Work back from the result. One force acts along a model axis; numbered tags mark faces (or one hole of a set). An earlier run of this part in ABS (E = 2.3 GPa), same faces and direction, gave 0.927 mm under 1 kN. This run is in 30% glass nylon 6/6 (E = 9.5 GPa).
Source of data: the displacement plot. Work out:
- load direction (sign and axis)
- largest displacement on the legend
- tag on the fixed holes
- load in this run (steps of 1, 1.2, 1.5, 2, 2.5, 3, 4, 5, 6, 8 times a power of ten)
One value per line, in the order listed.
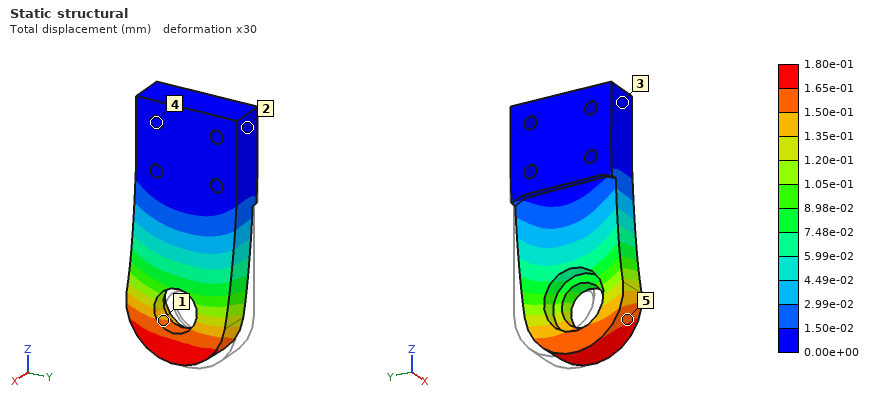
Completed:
-Y
1.80e-01 mm
4
800 N
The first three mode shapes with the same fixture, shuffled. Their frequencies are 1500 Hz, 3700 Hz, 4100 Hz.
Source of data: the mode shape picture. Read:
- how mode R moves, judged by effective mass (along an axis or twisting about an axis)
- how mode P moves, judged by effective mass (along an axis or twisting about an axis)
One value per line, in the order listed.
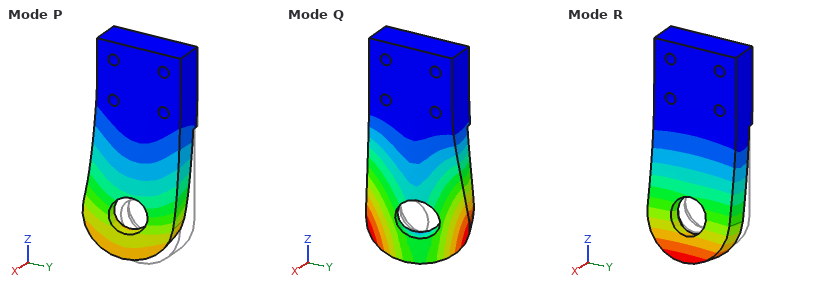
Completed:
along X
along Y
